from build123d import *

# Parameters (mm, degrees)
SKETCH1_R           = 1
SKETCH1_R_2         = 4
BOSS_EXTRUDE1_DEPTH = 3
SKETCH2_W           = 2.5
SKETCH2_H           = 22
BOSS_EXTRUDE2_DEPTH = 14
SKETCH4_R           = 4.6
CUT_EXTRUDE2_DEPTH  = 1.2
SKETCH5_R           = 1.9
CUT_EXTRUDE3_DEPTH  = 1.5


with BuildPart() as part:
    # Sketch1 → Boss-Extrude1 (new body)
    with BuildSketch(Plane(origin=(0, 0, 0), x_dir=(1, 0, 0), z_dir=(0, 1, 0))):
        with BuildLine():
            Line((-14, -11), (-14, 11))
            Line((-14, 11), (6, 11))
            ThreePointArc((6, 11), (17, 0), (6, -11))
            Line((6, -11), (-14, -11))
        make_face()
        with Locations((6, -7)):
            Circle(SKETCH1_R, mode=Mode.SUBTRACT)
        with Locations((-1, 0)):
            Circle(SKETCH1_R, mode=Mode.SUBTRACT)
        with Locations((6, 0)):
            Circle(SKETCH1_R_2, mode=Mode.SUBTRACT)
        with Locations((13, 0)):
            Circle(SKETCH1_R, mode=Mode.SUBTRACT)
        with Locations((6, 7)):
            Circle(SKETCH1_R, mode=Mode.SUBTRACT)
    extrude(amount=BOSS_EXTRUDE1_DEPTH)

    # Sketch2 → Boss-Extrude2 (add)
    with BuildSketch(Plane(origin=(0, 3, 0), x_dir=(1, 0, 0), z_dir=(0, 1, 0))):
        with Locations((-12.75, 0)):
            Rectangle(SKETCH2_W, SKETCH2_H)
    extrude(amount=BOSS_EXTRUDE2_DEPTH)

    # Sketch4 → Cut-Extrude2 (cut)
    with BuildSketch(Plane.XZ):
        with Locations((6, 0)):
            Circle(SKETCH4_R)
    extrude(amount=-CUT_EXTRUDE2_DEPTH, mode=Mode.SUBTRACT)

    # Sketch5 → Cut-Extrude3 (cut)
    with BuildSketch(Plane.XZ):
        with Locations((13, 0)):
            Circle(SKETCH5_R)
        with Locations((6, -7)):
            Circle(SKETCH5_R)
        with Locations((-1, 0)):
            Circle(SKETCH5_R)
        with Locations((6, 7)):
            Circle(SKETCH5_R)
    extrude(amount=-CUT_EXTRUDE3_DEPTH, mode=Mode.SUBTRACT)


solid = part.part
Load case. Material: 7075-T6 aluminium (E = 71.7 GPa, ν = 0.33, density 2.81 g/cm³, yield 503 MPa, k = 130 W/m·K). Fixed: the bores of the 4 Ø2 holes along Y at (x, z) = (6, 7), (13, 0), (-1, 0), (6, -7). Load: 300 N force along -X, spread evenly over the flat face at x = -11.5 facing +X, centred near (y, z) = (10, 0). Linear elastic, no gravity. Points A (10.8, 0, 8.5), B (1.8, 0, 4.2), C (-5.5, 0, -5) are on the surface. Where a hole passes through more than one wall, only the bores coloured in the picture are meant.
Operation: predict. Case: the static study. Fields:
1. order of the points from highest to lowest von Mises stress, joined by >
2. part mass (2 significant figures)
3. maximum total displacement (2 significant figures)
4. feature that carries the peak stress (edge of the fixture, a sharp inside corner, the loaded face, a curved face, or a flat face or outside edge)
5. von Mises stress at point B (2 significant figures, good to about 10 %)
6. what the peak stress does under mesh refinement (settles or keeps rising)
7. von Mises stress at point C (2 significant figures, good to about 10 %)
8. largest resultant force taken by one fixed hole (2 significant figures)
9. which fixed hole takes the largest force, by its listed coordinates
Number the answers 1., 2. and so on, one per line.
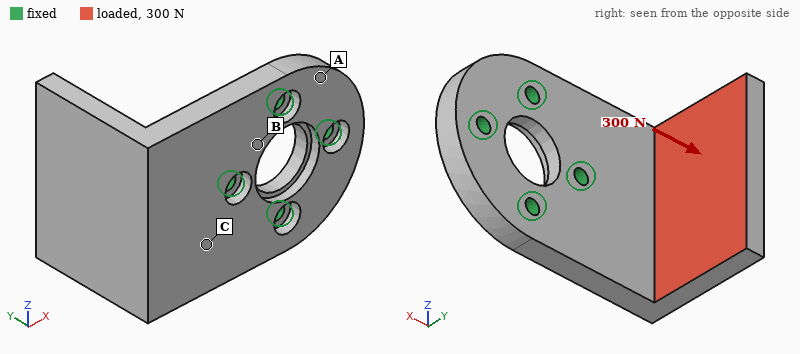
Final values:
1. C > B > A
2. 6.8 g
3. 0.23 mm
4. edge of the fixture
5. 39 MPa
6. keeps rising
7. 70 MPa
8. 470 N
9. (-1, 0)
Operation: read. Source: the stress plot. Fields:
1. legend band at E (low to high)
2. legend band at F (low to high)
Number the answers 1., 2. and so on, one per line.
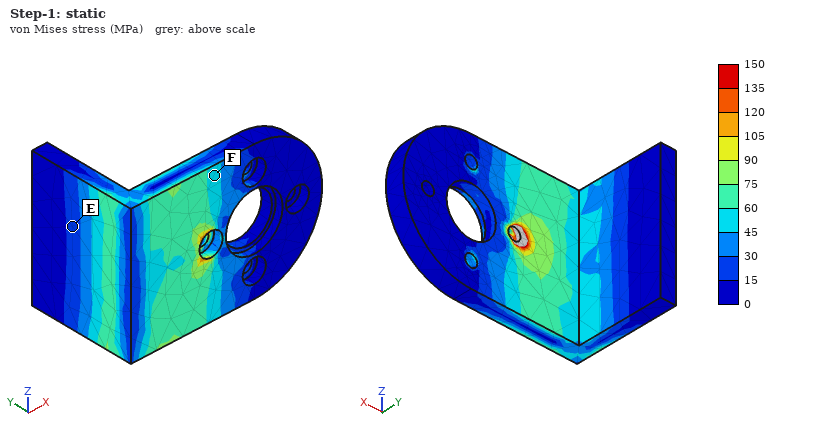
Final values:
1. 15 to 30 MPa
2. 45 to 60 MPa
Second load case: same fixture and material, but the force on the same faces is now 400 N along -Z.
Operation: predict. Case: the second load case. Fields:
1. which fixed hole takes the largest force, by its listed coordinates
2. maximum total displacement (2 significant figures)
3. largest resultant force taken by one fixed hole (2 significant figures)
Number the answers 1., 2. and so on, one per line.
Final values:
1. (-1, 0)
2. 0.20 mm
3. 520 N
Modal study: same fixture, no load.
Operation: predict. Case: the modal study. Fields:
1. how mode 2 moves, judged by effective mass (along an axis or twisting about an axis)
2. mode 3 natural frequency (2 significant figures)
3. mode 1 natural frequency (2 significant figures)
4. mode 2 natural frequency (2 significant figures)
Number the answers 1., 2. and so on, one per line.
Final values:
1. along Z
2. 9200 Hz
3. 3900 Hz
4. 5100 Hz
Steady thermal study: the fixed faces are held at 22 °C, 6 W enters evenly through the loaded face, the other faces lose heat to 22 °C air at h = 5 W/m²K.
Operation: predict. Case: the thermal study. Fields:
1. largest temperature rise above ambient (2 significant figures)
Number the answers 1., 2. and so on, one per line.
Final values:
1. 17 K
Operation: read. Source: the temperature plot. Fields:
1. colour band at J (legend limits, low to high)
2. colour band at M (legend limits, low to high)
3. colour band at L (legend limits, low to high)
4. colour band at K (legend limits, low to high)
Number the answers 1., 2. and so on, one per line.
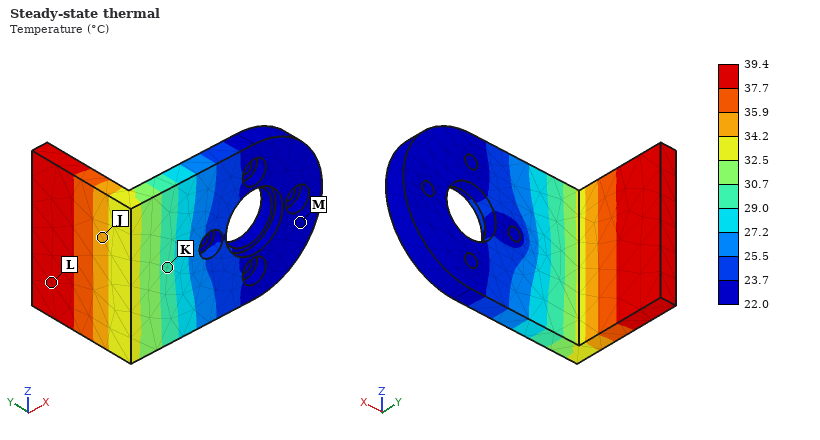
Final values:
1. 34.2 to 35.9 °C
2. 22.0 to 23.7 °C
3. 37.7 to 39.4 °C
4. 29.0 to 30.7 °C
